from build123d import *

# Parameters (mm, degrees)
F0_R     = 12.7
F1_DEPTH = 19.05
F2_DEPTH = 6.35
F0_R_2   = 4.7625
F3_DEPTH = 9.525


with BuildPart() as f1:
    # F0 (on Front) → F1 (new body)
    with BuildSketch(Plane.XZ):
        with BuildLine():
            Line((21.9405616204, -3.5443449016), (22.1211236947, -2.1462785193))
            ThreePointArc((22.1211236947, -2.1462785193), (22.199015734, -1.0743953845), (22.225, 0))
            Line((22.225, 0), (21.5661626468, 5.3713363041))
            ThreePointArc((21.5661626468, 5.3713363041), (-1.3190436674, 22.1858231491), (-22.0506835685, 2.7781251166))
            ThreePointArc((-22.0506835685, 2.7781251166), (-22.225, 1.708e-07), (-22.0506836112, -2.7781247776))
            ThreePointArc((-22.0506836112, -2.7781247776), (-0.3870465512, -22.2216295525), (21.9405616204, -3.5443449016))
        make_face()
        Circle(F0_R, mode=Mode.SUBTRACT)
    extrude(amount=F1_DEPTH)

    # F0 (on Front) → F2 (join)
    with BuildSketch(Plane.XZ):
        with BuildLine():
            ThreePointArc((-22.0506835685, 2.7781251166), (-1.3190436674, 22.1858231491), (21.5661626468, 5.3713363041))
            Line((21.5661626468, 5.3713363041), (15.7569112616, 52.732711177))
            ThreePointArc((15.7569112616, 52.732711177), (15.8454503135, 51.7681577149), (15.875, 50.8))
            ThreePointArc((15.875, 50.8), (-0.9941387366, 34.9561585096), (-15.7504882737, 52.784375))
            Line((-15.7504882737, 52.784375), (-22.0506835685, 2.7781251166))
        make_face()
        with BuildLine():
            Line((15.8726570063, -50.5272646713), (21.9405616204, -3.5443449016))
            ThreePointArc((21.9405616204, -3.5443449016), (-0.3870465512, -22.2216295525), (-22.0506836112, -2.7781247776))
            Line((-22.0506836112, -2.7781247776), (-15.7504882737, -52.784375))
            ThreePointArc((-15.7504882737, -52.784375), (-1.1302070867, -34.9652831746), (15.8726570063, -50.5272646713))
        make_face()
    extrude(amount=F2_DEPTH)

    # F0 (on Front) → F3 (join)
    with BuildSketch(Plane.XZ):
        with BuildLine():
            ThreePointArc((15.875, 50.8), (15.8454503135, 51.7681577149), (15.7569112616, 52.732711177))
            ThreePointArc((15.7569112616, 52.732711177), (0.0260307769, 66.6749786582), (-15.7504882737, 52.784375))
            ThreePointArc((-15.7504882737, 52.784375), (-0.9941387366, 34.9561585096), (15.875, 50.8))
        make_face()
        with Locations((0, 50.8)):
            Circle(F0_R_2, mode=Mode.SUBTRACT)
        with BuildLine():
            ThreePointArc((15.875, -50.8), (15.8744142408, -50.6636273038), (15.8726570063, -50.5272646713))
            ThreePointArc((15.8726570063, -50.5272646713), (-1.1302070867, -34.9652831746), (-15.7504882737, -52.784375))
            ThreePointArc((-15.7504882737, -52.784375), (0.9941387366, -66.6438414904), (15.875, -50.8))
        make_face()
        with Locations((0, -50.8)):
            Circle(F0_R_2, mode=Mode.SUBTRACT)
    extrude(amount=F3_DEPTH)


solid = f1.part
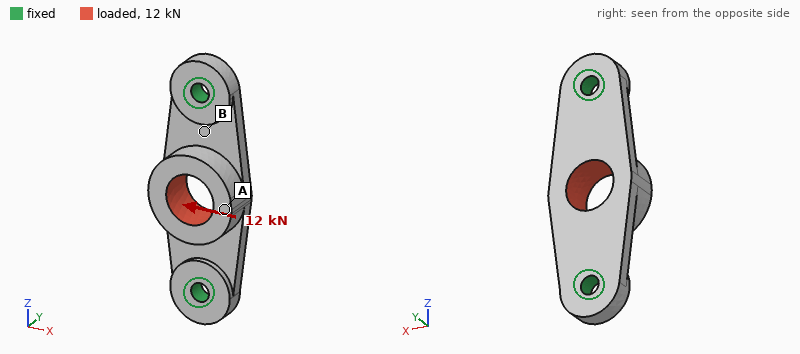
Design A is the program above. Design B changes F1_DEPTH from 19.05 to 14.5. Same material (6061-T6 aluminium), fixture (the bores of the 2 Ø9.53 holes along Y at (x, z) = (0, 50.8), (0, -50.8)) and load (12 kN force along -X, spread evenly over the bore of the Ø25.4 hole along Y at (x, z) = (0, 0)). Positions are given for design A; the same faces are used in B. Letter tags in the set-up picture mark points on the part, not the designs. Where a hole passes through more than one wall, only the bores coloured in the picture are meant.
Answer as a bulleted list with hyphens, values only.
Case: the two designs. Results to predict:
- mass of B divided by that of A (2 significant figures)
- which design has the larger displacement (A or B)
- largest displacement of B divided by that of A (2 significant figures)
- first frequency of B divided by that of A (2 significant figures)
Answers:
- 0.89
- A
- 0.66
- 1.1
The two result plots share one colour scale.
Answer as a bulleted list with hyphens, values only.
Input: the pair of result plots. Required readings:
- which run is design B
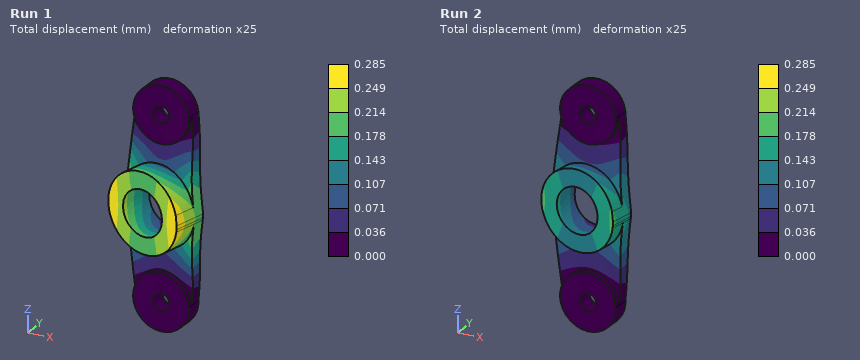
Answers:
- Run 2
